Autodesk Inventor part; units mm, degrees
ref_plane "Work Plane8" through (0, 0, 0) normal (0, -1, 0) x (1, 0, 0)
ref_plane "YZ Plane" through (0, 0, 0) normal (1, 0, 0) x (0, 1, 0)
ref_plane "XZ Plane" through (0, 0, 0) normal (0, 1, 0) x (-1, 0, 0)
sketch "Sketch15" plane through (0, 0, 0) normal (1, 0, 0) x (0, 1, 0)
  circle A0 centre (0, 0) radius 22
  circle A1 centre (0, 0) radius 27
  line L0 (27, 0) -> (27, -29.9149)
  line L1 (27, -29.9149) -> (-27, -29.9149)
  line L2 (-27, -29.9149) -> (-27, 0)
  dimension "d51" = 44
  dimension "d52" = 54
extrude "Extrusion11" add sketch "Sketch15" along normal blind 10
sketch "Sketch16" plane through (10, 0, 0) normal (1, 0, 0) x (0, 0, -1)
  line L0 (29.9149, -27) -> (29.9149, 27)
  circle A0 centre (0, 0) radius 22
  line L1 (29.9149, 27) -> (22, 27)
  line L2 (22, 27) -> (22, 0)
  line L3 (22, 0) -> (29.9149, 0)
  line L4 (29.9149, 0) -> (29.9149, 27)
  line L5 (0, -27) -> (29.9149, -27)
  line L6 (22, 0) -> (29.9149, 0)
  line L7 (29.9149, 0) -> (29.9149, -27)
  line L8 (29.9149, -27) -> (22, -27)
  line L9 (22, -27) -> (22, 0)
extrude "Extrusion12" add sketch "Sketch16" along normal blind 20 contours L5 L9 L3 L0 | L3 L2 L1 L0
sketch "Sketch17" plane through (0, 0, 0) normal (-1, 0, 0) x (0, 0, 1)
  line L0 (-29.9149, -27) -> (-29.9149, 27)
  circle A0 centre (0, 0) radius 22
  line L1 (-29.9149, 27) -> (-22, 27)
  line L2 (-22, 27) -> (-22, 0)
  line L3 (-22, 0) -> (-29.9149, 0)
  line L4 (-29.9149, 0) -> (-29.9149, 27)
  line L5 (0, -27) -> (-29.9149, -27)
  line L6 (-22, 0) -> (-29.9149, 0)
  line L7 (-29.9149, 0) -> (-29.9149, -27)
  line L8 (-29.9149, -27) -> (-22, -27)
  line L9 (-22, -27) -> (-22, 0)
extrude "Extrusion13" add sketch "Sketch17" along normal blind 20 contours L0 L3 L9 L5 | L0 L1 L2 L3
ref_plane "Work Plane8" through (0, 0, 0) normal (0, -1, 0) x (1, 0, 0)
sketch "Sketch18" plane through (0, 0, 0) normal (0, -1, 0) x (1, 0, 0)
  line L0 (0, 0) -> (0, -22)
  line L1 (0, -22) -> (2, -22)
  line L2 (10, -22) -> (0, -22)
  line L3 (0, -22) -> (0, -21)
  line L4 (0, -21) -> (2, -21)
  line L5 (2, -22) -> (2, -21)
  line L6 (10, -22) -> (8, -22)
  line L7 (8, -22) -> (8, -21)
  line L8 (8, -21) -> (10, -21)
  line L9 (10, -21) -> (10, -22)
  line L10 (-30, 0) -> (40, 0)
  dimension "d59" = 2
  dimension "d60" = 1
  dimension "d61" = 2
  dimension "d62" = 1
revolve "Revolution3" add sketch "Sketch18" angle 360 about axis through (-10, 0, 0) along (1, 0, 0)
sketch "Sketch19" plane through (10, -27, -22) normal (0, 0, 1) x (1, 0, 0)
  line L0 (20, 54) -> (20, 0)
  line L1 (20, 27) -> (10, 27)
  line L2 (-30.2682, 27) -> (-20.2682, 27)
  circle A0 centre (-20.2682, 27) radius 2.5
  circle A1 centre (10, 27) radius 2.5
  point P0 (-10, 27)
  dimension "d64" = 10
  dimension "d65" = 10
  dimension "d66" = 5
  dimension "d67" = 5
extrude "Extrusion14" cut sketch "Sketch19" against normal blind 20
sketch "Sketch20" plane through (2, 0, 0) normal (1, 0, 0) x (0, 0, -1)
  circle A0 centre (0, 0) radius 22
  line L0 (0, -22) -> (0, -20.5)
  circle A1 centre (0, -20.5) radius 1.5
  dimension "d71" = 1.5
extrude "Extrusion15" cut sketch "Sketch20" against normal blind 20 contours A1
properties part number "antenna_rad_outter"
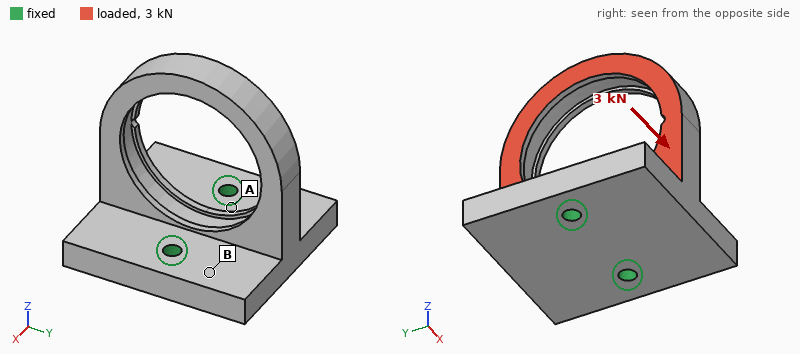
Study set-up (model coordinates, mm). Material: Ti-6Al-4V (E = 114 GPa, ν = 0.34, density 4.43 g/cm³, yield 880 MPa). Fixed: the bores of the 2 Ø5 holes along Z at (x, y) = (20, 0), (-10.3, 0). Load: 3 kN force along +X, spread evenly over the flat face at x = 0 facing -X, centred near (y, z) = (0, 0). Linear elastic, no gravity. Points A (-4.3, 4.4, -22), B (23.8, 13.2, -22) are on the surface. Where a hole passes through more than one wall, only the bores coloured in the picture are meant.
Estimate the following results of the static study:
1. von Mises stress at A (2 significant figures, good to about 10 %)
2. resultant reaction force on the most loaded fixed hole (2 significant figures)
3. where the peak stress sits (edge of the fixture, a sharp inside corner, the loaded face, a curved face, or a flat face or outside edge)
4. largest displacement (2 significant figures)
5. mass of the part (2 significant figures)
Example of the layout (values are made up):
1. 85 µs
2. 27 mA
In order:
1. 35 MPa
2. 3.0 kN
3. a curved face
4. 0.41 mm
5. 130 g
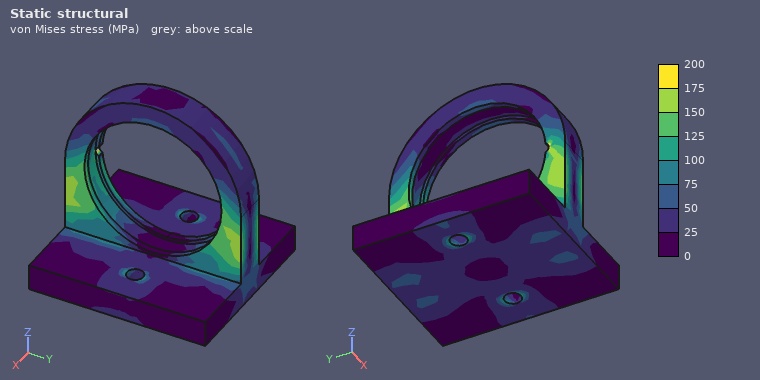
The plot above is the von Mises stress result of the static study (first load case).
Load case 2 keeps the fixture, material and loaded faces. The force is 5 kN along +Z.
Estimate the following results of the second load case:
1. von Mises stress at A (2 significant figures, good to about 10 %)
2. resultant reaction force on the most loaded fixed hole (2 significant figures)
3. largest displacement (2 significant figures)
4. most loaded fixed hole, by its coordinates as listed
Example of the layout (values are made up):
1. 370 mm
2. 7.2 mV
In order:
1. 73 MPa
2. 3.3 kN
3. 0.22 mm
4. (-10.3, 0)
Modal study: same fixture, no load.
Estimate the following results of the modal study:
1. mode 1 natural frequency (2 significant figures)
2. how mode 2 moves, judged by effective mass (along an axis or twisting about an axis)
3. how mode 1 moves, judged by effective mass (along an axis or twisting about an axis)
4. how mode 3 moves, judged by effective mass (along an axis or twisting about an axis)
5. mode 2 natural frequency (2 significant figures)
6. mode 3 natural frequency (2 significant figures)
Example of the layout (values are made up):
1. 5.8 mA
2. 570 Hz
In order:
1. 2700 Hz
2. along Y
3. along X
4. along Z
5. 2900 Hz
6. 5600 Hz
